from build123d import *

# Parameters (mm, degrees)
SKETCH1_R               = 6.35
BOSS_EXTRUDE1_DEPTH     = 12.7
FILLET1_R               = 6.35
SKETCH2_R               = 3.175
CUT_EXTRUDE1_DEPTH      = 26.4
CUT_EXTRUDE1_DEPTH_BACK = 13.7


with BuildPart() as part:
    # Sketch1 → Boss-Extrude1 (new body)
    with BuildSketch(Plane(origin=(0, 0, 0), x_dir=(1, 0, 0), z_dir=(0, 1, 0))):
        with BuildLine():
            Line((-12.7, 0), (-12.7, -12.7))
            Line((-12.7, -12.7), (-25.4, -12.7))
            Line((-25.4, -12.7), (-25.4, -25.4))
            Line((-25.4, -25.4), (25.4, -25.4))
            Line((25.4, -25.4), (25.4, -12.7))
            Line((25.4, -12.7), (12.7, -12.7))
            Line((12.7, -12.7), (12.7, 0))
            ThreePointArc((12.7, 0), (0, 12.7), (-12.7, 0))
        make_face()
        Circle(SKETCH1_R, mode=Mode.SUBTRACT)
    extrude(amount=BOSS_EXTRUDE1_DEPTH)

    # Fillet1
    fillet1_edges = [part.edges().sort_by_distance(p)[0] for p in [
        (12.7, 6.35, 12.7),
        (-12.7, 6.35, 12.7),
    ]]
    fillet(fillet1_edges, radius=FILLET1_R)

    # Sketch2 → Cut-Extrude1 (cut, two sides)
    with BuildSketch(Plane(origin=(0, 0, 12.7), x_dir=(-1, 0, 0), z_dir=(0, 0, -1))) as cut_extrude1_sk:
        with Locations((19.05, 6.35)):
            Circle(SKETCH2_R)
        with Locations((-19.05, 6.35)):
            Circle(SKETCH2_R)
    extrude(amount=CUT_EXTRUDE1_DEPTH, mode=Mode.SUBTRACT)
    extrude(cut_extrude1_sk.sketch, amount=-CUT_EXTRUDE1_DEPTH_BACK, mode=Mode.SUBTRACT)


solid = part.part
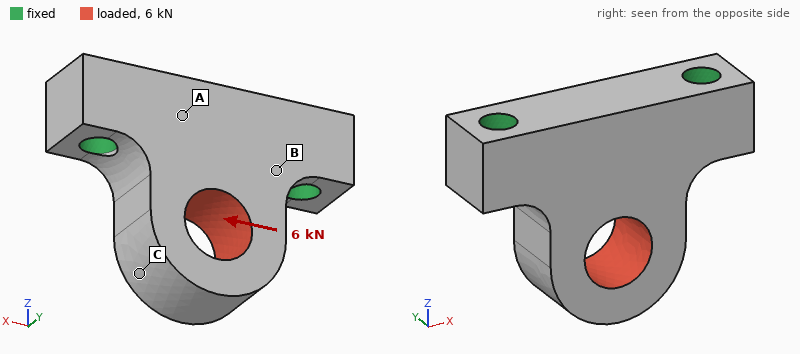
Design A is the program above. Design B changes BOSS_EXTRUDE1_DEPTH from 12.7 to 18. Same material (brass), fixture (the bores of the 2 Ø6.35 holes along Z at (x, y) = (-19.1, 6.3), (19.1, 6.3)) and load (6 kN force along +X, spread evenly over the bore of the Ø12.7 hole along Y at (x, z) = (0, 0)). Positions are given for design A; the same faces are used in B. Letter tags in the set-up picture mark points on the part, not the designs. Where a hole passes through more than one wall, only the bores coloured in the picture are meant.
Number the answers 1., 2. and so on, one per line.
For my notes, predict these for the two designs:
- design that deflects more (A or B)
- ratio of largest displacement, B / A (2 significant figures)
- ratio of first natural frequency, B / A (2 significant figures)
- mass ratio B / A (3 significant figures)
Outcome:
1. A
2. 0.74
3. 1.1
4. 1.44
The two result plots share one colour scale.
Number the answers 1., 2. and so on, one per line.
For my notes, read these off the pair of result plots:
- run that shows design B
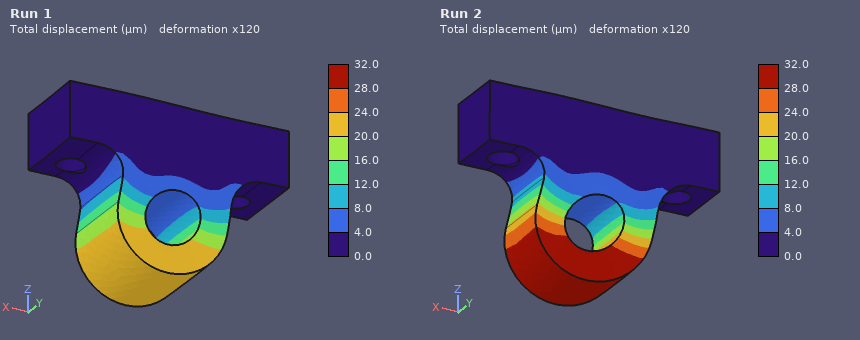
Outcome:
1. Run 1
